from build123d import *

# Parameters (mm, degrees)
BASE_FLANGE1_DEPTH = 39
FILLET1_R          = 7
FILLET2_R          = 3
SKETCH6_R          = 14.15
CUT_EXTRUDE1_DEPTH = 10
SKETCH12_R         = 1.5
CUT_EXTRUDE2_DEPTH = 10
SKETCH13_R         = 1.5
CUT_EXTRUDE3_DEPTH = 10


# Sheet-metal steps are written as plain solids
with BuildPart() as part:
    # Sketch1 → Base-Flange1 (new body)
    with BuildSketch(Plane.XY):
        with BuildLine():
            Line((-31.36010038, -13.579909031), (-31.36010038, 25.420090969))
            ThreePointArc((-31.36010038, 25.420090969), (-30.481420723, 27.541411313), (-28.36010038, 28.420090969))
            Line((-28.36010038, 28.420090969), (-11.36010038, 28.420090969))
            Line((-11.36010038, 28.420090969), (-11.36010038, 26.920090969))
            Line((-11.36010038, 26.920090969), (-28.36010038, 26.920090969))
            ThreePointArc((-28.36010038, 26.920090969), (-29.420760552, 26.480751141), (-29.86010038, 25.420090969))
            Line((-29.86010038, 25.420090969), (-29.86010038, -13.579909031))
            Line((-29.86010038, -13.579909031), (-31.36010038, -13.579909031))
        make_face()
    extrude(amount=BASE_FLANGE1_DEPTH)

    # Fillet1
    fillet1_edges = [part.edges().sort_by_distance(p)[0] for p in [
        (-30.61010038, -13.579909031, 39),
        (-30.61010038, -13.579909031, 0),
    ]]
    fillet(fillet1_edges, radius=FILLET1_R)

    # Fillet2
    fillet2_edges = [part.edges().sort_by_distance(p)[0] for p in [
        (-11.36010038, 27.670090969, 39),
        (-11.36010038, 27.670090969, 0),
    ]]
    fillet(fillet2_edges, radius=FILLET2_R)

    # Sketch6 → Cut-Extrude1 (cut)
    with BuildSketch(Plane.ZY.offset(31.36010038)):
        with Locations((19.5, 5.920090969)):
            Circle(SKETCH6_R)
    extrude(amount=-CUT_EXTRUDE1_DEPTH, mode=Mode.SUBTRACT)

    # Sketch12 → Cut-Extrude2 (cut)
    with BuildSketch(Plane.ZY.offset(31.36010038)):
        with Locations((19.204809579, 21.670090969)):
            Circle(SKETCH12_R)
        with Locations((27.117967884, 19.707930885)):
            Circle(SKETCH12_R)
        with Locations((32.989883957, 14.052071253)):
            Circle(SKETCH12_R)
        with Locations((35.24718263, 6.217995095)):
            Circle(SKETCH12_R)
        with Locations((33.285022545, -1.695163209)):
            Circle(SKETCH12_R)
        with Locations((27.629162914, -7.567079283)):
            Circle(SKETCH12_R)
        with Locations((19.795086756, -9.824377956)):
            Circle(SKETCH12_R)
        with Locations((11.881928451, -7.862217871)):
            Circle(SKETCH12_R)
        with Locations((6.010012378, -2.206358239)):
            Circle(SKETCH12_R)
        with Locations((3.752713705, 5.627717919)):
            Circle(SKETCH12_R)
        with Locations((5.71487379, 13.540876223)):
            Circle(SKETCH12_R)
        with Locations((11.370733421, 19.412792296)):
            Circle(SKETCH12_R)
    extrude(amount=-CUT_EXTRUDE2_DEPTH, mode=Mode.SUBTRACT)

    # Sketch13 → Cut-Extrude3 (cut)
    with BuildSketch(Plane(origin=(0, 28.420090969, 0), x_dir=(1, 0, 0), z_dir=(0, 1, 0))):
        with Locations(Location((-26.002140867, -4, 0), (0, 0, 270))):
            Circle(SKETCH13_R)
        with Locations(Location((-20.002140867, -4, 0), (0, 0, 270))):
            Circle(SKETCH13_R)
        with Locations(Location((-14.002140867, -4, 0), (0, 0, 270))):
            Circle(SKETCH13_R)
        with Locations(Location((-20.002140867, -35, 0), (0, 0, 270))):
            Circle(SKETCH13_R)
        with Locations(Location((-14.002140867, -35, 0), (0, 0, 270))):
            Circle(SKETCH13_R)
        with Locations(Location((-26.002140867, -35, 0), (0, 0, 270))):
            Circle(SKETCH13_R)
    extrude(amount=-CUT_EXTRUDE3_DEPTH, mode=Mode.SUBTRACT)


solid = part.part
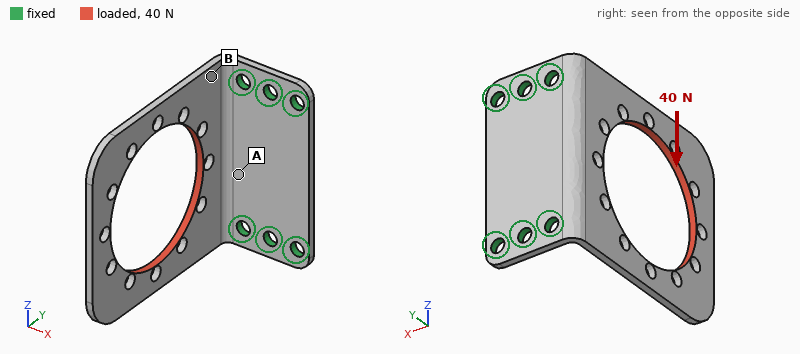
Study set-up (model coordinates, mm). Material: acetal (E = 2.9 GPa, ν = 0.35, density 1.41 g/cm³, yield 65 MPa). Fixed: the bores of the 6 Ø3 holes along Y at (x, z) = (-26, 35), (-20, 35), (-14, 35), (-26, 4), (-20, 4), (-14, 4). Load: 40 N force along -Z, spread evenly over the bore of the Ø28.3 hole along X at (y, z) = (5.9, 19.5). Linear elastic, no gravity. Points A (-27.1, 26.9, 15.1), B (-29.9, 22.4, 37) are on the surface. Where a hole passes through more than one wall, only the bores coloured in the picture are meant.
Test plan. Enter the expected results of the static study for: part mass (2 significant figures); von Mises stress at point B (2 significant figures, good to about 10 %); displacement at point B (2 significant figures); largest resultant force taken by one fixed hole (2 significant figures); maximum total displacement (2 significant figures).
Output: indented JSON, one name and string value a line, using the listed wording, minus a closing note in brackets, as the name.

{
  "part mass": "3.3 g",
  "von Mises stress at point B": "6.2 MPa",
  "displacement at point B": "0.12 mm",
  "largest resultant force taken by one fixed hole": "32 N",
  "maximum total displacement": "0.60 mm"
}
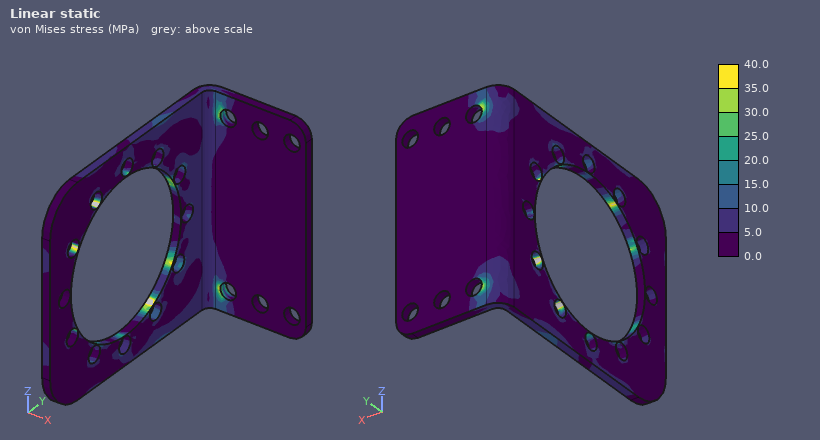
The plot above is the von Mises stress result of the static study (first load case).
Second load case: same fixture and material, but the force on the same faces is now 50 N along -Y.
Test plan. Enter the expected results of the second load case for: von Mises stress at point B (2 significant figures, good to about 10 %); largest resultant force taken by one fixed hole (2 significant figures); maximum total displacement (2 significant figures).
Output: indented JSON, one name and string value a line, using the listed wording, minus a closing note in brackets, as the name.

{
  "von Mises stress at point B": "3.4 MPa",
  "largest resultant force taken by one fixed hole": "28 N",
  "maximum total displacement": "0.69 mm"
}
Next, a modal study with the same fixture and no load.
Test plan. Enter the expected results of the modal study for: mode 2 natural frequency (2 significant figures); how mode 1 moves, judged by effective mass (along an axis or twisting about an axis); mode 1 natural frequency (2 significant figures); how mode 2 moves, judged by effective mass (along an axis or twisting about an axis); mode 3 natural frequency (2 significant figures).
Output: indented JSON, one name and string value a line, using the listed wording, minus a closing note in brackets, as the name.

{
  "mode 2 natural frequency": "390 Hz",
  "how mode 1 moves, judged by effective mass": "along X",
  "mode 1 natural frequency": "160 Hz",
  "how mode 2 moves, judged by effective mass": "twisting about Y",
  "mode 3 natural frequency": "970 Hz"
}
